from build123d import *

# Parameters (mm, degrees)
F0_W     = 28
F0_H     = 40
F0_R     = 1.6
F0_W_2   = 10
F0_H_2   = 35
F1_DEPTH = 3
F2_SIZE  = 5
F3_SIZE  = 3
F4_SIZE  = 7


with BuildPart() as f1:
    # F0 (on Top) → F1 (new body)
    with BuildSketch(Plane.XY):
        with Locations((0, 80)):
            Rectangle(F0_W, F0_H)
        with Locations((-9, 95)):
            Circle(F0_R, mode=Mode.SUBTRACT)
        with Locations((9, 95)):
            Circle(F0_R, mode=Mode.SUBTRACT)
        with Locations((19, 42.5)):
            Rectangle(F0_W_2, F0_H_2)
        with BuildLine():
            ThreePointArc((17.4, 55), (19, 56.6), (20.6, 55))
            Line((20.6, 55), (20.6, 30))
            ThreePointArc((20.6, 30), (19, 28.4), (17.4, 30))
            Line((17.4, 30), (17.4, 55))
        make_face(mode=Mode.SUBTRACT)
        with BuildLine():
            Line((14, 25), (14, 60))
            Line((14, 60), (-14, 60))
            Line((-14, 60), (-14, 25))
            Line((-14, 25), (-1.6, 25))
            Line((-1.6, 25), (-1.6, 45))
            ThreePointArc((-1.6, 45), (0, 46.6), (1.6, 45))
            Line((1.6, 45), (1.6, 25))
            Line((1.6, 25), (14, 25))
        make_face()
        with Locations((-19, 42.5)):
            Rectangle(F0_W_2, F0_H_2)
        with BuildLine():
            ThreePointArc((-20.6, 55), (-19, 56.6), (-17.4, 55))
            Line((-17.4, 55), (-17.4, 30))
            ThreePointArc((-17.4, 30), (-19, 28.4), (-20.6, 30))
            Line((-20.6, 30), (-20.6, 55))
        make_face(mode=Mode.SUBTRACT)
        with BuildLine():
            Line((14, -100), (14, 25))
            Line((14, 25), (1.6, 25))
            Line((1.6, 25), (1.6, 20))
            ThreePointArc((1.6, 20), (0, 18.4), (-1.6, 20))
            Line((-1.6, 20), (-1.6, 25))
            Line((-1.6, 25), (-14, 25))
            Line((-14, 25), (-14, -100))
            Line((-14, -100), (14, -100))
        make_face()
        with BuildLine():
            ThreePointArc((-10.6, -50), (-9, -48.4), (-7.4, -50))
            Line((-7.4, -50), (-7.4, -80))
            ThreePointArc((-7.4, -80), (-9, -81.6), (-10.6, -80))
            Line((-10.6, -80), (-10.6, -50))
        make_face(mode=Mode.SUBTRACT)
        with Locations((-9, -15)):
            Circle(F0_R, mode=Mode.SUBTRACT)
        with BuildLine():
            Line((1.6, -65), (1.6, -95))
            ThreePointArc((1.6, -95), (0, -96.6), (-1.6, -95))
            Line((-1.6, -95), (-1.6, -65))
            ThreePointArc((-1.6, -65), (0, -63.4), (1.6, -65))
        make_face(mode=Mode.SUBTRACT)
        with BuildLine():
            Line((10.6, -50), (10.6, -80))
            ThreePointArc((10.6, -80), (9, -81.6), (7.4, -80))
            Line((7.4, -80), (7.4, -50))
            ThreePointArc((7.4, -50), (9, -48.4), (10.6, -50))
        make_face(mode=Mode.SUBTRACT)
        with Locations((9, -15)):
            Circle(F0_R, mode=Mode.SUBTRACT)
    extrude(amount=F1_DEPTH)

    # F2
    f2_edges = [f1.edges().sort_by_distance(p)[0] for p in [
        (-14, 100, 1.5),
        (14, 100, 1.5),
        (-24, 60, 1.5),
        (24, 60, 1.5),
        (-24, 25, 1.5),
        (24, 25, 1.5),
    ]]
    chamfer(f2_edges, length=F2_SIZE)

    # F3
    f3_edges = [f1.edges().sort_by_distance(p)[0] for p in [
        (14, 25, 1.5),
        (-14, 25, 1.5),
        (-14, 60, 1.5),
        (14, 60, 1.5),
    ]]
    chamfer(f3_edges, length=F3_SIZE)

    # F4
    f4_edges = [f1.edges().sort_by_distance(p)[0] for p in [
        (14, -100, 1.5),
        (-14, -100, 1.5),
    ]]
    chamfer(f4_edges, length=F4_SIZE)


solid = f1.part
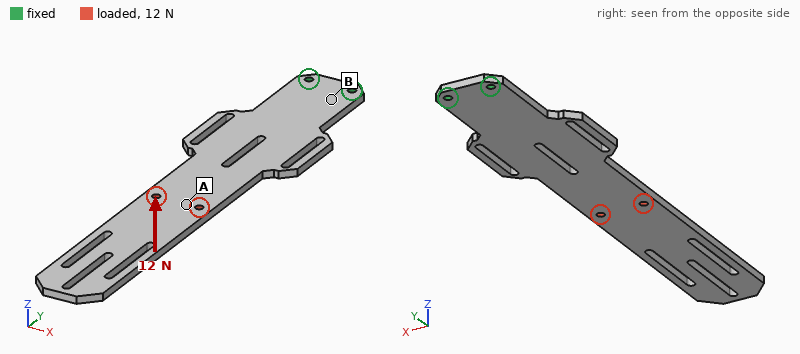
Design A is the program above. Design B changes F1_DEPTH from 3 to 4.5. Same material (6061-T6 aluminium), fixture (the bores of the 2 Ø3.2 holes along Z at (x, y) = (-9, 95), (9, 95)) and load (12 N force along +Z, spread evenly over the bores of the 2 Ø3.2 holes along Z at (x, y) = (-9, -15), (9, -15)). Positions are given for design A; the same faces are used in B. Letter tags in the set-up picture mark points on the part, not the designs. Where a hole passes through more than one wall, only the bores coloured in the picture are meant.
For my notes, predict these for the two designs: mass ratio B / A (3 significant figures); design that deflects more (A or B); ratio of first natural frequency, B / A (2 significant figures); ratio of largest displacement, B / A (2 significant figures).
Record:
1.50
A
1.5
0.30
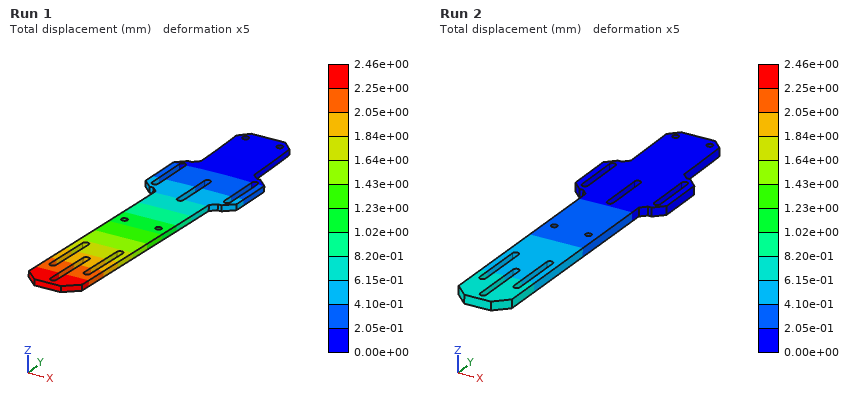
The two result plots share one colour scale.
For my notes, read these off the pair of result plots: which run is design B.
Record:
Run 2
